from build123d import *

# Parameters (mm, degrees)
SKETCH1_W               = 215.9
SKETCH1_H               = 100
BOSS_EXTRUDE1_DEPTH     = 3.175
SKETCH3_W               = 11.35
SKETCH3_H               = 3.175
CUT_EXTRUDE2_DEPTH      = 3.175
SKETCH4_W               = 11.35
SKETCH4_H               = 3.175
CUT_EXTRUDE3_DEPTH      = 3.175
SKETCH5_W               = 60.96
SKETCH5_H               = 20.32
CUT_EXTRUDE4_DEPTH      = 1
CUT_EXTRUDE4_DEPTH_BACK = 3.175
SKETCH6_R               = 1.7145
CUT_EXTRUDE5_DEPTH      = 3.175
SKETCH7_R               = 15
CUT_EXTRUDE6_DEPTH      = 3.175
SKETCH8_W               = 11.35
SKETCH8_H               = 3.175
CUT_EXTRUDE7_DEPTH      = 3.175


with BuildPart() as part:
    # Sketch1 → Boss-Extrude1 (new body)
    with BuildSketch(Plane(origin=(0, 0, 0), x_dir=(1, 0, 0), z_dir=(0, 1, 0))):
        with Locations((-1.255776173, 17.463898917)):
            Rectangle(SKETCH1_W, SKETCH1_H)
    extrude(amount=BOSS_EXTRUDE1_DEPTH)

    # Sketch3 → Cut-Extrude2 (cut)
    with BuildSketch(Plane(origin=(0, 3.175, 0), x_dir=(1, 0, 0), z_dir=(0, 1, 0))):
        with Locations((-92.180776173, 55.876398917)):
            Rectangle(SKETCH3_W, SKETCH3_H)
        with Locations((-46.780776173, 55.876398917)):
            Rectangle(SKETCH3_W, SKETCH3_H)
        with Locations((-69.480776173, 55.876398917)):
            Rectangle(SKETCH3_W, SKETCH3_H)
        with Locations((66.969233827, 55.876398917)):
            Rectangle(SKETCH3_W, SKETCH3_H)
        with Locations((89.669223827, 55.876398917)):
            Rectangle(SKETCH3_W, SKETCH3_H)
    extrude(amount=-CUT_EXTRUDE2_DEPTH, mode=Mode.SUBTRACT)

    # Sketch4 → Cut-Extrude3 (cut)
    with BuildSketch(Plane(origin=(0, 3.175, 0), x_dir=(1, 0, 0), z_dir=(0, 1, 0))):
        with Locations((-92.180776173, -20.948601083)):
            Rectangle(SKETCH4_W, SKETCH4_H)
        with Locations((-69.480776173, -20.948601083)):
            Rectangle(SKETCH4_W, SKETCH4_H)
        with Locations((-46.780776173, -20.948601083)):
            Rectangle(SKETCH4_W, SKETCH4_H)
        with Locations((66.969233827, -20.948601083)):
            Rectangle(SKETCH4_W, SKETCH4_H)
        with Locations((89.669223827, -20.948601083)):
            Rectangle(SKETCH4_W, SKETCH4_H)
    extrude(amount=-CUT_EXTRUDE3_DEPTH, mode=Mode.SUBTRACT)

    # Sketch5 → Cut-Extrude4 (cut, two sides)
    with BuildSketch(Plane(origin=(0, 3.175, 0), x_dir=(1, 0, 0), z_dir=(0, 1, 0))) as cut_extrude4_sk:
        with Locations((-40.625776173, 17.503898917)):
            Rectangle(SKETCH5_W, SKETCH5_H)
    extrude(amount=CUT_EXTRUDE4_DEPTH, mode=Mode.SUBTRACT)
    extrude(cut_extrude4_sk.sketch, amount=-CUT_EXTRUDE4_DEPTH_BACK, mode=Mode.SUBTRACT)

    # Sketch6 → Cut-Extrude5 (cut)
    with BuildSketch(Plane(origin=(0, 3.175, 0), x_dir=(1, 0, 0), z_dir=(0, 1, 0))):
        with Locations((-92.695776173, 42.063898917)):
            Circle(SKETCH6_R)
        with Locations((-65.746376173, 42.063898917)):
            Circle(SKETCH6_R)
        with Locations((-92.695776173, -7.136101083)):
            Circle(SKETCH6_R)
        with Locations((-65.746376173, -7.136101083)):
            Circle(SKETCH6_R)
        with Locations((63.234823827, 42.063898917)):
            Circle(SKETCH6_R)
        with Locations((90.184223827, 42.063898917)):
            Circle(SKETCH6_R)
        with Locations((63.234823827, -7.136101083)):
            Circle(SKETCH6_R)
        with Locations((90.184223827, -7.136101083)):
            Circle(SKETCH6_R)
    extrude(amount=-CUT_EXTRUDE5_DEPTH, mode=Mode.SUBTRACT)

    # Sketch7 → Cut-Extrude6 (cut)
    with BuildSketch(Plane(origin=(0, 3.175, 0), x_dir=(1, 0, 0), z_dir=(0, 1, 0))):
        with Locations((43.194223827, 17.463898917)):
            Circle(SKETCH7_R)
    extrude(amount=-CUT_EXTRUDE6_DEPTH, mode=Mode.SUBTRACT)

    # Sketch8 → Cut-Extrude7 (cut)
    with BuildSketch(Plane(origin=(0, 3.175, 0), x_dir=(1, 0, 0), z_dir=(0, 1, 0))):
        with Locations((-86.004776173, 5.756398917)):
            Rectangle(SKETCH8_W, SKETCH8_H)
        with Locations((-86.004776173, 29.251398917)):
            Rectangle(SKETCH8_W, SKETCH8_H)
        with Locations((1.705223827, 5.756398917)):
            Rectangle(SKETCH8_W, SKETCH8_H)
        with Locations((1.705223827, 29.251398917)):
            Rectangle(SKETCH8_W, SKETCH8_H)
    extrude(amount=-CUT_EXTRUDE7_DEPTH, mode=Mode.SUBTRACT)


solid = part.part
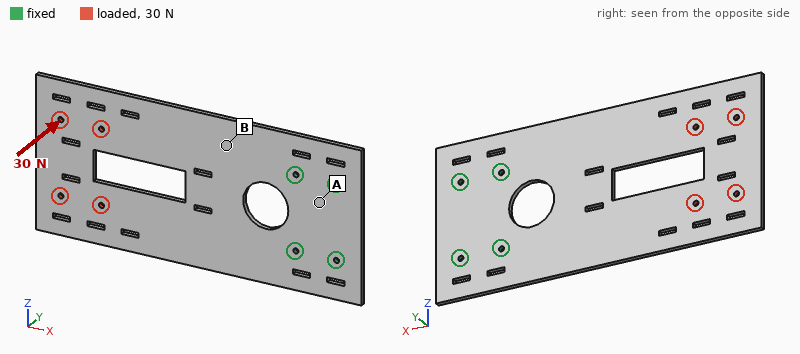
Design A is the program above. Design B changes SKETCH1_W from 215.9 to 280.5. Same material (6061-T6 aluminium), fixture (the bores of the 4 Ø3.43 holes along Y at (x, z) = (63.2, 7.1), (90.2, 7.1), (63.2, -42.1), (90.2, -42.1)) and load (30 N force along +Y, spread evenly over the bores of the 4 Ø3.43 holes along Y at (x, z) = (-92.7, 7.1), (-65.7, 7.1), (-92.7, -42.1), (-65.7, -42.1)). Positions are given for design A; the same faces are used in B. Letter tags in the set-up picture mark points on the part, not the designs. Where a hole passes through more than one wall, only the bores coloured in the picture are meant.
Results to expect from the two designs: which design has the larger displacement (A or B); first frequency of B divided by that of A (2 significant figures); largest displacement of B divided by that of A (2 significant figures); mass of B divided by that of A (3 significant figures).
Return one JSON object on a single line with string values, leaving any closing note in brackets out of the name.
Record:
{"which design has the larger displacement": "B", "first frequency of B divided by that of A": "0.69", "largest displacement of B divided by that of A": "1.3", "mass of B divided by that of A": "1.34"}
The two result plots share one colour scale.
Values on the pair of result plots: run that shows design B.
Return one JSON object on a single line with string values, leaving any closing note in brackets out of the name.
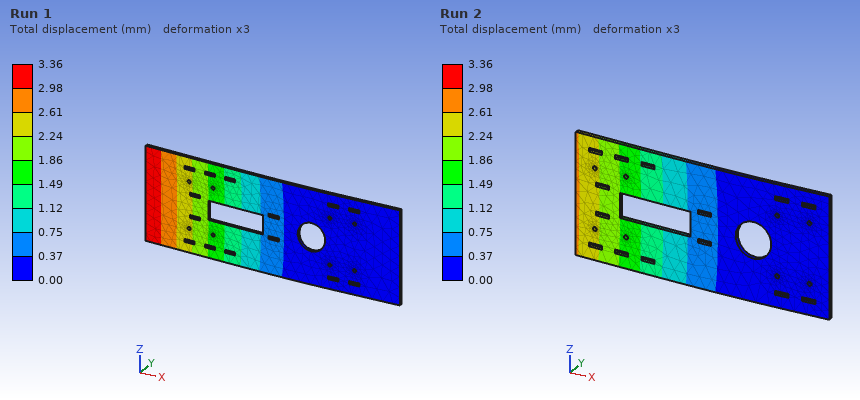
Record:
{"run that shows design B": "Run 1"}
